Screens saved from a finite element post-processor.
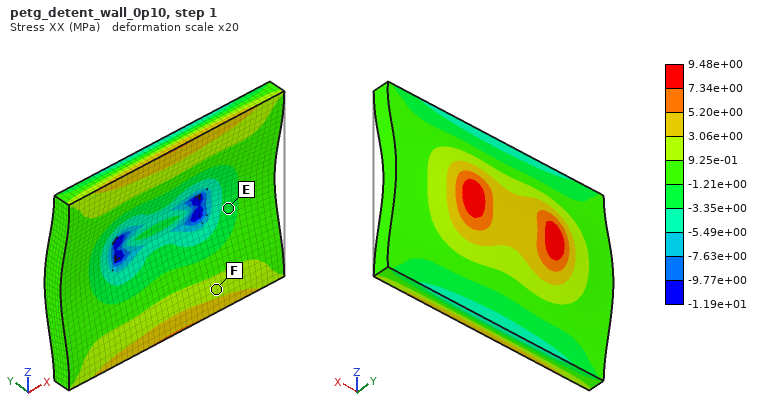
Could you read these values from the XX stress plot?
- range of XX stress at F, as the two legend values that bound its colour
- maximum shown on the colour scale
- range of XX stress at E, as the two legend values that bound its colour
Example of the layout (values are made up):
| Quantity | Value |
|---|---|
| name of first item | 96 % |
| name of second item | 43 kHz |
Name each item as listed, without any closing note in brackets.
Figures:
| Quantity | Value |
|---|---|
| range of XX stress at F, as the two legend values that bound its colour | 9.25e-01 to 3.06e+00 MPa |
| maximum shown on the colour scale | 9.48e+00 MPa |
| range of XX stress at E, as the two legend values that bound its colour | -3.35e+00 to -1.21e+00 MPa |
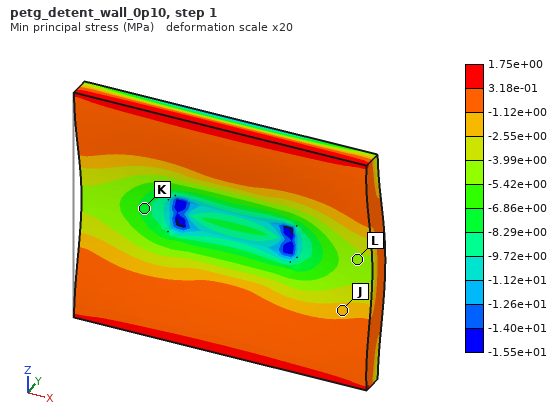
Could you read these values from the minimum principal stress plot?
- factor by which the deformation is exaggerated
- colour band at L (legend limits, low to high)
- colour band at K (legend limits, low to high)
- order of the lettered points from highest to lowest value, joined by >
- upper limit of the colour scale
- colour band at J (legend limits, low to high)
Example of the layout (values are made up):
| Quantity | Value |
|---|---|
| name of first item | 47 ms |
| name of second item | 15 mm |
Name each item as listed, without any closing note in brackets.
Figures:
| Quantity | Value |
|---|---|
| factor by which the deformation is exaggerated | 20 |
| colour band at L | -5.42e+00 to -3.99e+00 MPa |
| colour band at K | -8.29e+00 to -6.86e+00 MPa |
| order of the lettered points from highest to lowest value, joined by > | J > L > K |
| upper limit of the colour scale | 1.75e+00 MPa |
| colour band at J | -2.55e+00 to -1.12e+00 MPa |
